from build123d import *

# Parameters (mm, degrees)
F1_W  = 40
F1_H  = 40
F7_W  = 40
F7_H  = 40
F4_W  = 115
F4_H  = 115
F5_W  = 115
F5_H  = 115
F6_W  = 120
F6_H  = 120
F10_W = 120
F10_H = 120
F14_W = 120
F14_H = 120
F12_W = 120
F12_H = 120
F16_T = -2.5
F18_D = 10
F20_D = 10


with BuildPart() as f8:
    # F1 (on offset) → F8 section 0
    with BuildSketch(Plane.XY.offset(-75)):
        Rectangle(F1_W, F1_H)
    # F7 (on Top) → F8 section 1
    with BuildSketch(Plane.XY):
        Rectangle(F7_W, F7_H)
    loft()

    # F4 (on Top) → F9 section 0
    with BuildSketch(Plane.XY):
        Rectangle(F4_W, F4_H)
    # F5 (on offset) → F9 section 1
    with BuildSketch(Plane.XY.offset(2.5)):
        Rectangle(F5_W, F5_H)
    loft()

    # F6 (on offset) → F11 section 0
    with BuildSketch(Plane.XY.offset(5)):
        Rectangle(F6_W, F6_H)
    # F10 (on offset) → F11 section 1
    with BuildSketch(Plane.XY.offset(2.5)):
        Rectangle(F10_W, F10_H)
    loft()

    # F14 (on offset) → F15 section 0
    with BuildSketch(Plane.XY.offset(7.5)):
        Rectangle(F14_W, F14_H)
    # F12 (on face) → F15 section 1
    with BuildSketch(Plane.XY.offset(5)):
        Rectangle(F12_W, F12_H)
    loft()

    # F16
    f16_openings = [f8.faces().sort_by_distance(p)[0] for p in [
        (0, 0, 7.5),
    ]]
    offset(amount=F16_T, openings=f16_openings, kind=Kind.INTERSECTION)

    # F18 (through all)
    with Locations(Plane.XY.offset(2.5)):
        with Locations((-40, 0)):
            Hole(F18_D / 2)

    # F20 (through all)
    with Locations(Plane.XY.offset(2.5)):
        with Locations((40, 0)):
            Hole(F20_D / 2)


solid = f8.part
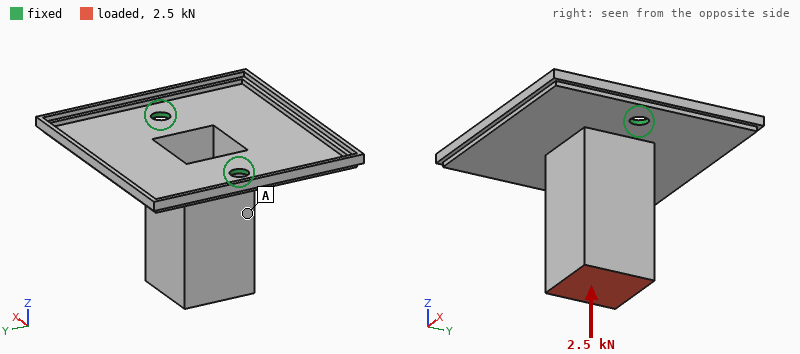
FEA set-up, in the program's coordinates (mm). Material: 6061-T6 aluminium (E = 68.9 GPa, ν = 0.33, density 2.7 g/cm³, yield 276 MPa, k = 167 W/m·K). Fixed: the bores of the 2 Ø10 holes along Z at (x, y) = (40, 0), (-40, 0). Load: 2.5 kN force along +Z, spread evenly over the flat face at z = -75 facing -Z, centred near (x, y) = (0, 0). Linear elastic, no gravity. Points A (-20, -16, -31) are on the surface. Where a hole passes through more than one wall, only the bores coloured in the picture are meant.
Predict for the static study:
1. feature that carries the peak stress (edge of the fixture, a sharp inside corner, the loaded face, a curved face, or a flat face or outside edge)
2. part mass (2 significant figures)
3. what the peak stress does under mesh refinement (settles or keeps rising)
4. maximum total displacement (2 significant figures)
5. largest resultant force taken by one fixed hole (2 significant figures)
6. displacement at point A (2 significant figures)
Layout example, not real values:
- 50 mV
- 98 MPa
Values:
- edge of the fixture
- 190 g
- keeps rising
- 0.31 mm
- 1.5 kN
- 0.24 mm
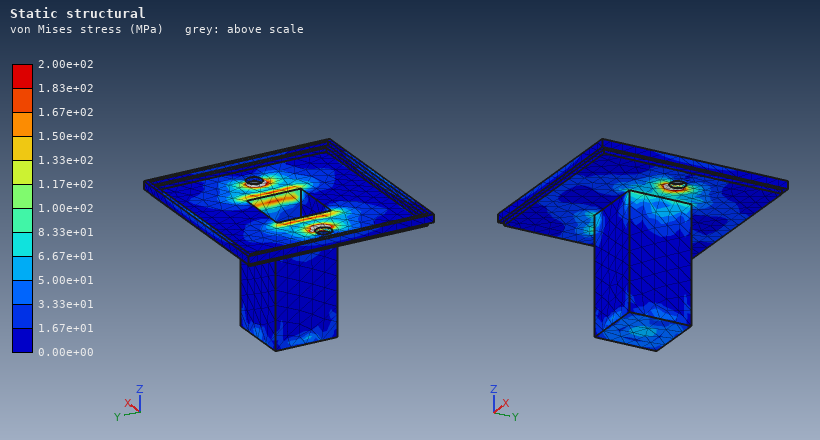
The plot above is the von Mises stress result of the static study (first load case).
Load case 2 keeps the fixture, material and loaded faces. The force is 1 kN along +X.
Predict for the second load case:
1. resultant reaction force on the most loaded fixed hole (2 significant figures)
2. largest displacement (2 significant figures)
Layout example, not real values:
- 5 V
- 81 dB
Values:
- 1.3 kN
- 0.68 mm
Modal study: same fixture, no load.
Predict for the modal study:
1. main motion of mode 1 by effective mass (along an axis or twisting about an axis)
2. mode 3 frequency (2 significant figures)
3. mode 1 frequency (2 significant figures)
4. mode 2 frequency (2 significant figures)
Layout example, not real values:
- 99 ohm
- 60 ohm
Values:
- along Y
- 980 Hz
- 400 Hz
- 960 Hz
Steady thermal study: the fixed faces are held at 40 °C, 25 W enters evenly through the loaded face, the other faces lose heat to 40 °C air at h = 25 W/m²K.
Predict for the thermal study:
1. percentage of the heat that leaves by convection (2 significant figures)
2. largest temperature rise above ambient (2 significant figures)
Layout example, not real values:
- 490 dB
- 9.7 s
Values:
- 52 %
- 32 K
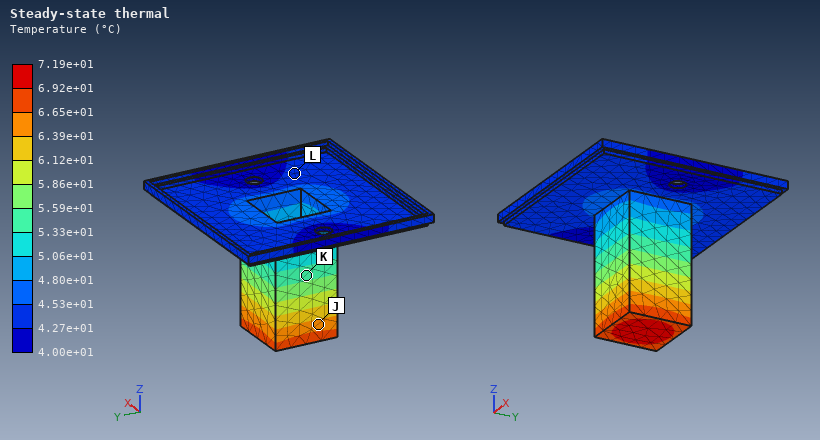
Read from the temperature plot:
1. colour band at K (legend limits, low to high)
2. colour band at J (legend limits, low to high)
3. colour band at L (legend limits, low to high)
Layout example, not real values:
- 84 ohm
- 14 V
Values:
- 5.33e+01 to 5.59e+01 °C
- 6.39e+01 to 6.65e+01 °C
- 4.27e+01 to 4.53e+01 °C
